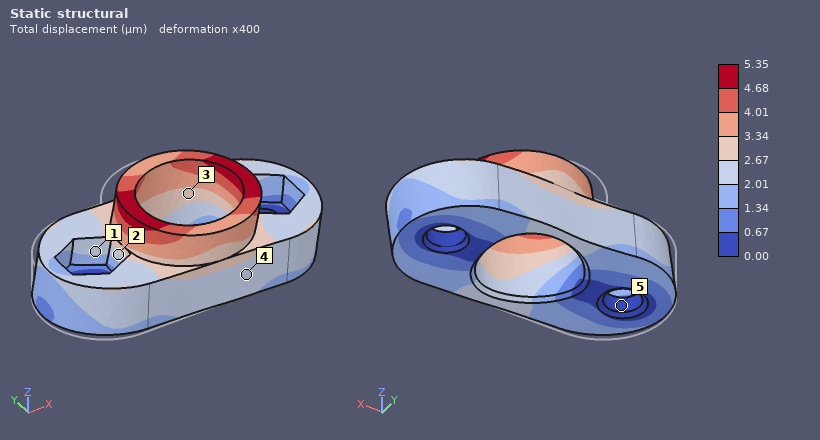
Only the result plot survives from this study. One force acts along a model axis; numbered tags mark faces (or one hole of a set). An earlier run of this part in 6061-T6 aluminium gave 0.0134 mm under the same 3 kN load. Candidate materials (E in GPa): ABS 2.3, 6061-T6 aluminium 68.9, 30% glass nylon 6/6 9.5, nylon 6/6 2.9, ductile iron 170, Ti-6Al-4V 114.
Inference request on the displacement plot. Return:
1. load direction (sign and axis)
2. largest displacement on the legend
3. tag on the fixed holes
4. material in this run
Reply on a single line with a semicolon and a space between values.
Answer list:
+X; 5.35 µm; 5; ductile iron
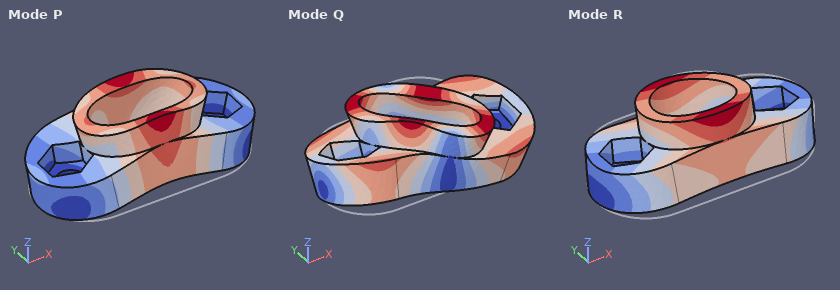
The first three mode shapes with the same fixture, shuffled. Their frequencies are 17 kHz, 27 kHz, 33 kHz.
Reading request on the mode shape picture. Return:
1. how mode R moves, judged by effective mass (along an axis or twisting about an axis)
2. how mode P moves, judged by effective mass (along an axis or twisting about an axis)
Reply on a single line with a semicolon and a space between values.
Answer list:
along Y; along Z
